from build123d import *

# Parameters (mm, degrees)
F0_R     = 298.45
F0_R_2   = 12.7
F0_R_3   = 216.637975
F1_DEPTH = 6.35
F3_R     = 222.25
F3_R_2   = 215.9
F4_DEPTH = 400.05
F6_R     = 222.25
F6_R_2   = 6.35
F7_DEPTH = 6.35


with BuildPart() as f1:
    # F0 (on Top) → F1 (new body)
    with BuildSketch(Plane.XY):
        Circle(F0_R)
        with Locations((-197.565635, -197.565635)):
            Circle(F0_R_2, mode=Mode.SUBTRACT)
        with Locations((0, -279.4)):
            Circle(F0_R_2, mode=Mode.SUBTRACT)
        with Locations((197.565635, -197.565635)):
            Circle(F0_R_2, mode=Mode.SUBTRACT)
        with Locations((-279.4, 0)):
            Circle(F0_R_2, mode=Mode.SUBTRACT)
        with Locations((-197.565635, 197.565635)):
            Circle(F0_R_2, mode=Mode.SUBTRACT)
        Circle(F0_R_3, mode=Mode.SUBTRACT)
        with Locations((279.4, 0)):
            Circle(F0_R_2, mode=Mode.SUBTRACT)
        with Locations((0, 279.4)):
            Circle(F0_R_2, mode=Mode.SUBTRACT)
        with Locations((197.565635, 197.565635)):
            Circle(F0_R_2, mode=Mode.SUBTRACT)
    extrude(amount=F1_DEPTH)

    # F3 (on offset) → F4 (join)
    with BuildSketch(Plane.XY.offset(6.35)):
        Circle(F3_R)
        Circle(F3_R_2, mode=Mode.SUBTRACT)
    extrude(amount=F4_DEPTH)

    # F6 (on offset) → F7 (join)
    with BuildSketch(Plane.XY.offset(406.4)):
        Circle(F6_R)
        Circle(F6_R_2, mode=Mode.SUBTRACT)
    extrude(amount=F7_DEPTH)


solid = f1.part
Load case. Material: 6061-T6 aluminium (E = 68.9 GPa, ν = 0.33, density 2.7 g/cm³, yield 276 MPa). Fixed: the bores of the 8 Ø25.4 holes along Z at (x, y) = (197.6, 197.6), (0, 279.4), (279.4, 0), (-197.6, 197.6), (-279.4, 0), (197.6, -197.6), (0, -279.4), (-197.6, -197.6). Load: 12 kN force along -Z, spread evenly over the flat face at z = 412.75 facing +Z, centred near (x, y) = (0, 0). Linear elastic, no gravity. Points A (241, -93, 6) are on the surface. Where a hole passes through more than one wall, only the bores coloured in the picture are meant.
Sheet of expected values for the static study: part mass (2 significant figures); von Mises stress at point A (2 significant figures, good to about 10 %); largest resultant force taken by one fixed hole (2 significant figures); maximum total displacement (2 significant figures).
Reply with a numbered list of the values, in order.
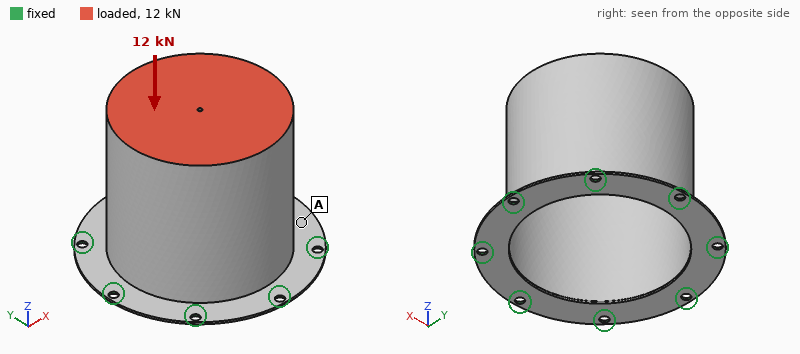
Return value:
1. 14 kg
2. 7.0 MPa
3. 1.9 kN
4. 2.2 mm
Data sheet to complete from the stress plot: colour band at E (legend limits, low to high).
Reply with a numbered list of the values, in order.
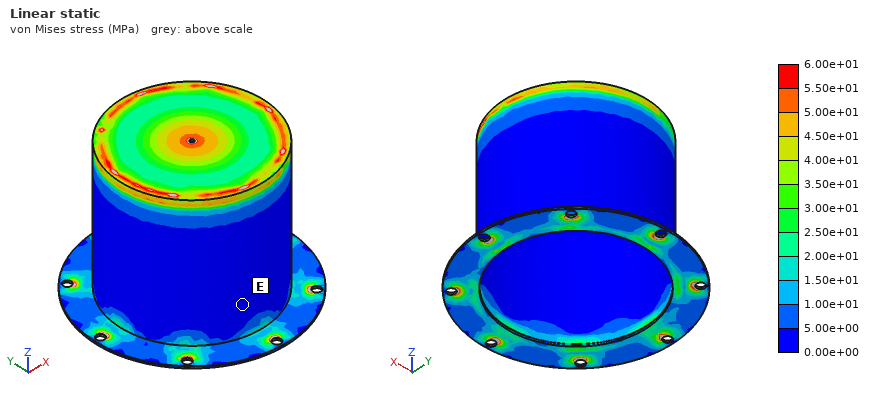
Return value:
1. 0.00e+00 to 5.00e+00 MPa
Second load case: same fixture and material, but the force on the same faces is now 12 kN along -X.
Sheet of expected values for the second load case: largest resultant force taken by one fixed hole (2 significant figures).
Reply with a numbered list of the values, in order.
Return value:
1. 6.2 kN
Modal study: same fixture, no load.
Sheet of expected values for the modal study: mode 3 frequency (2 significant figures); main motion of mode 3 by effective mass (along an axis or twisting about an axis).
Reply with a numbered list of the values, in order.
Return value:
1. 280 Hz
2. along Z
